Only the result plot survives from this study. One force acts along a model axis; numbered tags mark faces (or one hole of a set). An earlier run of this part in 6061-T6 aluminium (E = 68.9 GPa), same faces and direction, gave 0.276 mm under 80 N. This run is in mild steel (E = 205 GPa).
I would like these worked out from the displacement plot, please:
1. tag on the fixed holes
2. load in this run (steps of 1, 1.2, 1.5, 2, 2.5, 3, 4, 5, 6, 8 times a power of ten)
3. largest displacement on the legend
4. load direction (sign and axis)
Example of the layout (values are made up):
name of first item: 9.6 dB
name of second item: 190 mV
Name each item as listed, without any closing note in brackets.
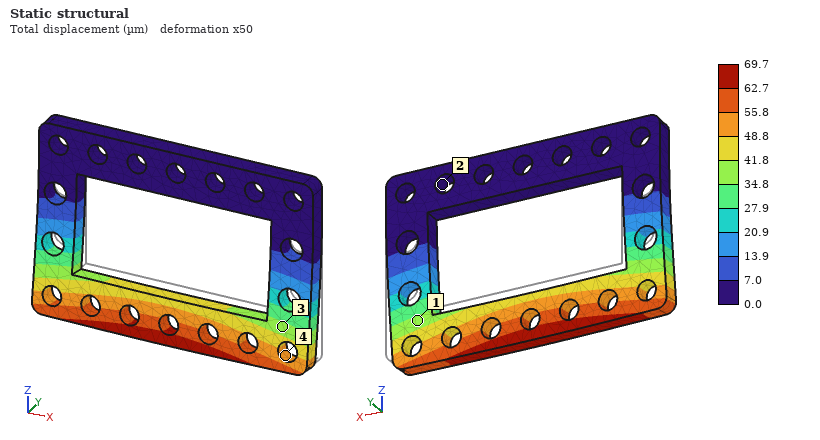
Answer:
tag on the fixed holes: 2
load in this run: 60 N
largest displacement on the legend: 69.7 µm
load direction: -Y
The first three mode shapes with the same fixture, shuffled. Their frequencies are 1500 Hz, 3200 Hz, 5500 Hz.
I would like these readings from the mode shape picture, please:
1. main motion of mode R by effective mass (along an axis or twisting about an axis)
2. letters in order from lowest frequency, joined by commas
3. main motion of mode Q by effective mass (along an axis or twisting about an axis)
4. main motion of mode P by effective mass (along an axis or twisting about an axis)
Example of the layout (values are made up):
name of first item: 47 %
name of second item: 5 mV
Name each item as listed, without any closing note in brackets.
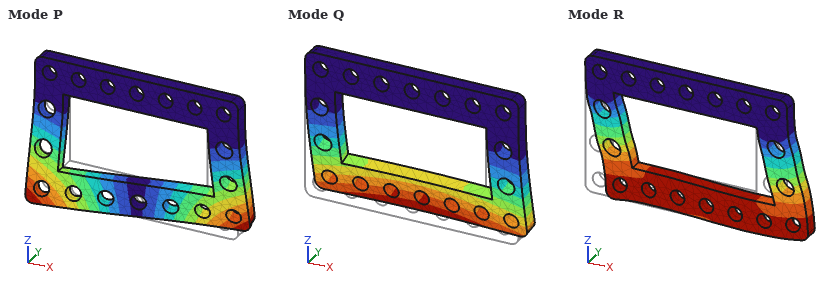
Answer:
main motion of mode R by effective mass: along X
letters in order from lowest frequency, joined by commas: Q, P, R
main motion of mode Q by effective mass: along Y
main motion of mode P by effective mass: twisting about Z
